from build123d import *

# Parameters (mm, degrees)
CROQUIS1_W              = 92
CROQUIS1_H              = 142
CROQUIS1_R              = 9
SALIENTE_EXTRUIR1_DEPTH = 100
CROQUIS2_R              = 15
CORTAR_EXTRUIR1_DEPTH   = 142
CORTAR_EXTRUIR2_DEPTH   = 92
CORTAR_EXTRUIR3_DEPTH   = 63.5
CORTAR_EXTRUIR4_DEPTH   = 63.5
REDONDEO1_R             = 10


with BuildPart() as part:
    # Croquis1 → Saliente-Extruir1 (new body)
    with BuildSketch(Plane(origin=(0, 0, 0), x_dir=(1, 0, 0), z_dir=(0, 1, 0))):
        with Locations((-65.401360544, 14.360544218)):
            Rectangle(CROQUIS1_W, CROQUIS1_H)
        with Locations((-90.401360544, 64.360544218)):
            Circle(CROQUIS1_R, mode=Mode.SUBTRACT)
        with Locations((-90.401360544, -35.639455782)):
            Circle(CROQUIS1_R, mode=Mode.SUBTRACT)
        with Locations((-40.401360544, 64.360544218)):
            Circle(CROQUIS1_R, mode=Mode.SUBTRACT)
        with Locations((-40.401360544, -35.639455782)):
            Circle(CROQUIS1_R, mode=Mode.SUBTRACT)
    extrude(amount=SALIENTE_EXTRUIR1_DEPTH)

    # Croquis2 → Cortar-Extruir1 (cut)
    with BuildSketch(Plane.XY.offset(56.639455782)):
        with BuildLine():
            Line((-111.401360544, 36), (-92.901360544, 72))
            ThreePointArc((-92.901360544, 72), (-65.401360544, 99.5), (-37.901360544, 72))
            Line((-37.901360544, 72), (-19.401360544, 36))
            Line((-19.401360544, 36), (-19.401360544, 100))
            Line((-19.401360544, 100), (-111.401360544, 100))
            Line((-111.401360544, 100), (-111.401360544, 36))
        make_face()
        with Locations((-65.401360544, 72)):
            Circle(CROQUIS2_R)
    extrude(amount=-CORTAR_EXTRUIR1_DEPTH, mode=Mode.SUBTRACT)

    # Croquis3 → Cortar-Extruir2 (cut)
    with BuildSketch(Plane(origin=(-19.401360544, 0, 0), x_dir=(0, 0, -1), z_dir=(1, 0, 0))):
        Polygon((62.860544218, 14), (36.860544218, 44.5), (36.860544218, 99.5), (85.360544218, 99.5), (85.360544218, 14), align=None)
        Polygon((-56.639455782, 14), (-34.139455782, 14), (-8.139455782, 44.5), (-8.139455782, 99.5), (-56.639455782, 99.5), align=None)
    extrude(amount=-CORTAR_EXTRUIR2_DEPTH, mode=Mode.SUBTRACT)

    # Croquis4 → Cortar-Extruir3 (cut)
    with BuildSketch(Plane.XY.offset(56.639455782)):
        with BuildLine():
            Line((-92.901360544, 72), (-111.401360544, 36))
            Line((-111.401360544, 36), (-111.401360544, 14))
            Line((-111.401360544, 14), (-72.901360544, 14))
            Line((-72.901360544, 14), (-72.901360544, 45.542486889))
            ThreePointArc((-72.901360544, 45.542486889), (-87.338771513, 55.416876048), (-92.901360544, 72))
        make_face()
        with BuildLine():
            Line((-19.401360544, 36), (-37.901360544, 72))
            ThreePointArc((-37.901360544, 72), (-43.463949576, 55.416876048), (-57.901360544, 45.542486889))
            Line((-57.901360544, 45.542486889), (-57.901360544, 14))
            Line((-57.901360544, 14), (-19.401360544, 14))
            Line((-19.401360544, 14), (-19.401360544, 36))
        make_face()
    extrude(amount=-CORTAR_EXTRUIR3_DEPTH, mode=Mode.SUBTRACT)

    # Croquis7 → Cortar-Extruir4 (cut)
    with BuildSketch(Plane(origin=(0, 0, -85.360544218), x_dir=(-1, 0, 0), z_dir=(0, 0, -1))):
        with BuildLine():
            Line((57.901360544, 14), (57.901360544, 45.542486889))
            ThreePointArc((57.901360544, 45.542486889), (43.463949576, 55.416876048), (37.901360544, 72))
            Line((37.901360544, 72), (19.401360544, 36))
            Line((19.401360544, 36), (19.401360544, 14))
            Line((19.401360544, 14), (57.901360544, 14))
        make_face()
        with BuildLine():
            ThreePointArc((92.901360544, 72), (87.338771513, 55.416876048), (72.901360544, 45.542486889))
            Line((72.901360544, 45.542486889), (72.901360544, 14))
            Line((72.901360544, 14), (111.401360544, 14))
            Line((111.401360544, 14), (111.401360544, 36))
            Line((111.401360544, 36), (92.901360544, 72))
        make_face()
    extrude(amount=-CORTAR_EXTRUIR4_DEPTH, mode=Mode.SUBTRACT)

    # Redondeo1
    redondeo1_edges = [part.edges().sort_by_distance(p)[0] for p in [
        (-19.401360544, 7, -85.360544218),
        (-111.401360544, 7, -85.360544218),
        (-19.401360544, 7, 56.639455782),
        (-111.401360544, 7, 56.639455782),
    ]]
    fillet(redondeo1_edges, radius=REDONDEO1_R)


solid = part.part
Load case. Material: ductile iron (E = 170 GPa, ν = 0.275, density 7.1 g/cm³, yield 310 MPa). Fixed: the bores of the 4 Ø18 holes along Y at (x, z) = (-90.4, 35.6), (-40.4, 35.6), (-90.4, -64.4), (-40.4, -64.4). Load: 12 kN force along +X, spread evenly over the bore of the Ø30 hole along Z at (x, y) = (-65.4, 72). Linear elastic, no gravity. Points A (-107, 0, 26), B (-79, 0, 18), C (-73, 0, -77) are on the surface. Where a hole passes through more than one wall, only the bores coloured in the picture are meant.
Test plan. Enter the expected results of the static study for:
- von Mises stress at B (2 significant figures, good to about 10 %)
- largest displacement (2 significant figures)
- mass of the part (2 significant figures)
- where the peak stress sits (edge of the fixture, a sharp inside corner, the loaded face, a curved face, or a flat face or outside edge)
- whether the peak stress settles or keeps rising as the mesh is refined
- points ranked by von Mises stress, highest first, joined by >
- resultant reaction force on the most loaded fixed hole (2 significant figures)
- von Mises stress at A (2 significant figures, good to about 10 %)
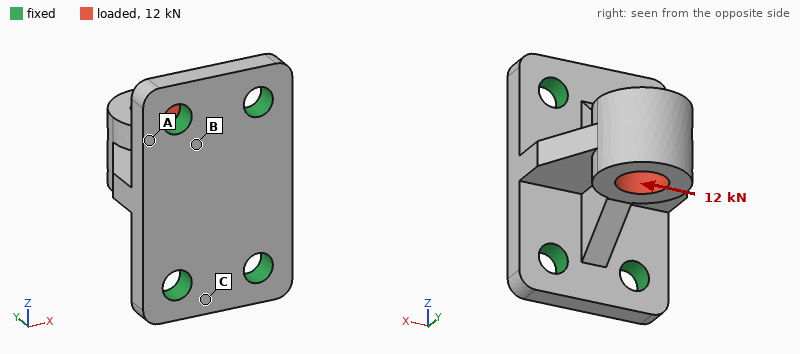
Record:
26 MPa
96 µm
2.3 kg
edge of the fixture
keeps rising
A > B > C
7.9 kN
46 MPa
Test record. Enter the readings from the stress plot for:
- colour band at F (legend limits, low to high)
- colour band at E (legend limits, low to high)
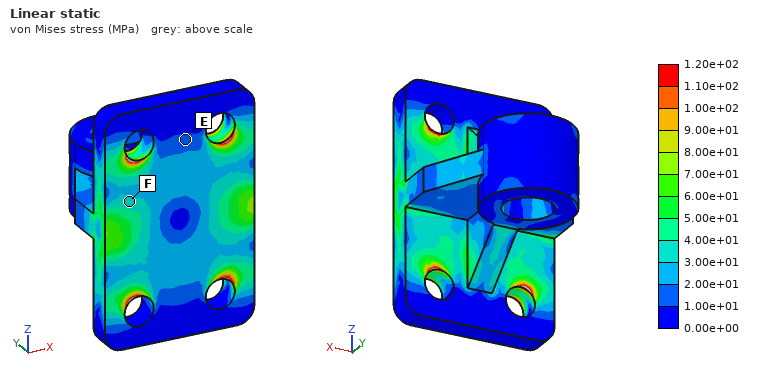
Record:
3.00e+01 to 4.00e+01 MPa
1.00e+01 to 2.00e+01 MPa
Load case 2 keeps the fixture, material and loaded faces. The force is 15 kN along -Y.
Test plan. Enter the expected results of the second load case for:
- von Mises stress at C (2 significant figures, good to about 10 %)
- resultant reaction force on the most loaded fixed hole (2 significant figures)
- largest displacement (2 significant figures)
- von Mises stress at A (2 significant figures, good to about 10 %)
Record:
5.9 MPa
4.1 kN
14 µm
12 MPa
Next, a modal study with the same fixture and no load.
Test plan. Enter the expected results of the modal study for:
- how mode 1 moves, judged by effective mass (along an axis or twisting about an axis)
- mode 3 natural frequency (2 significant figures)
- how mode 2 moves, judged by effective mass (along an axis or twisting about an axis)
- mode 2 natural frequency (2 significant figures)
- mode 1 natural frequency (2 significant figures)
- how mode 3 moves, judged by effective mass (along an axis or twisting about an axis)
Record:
along X
5400 Hz
along Z
3500 Hz
2400 Hz
along Y
